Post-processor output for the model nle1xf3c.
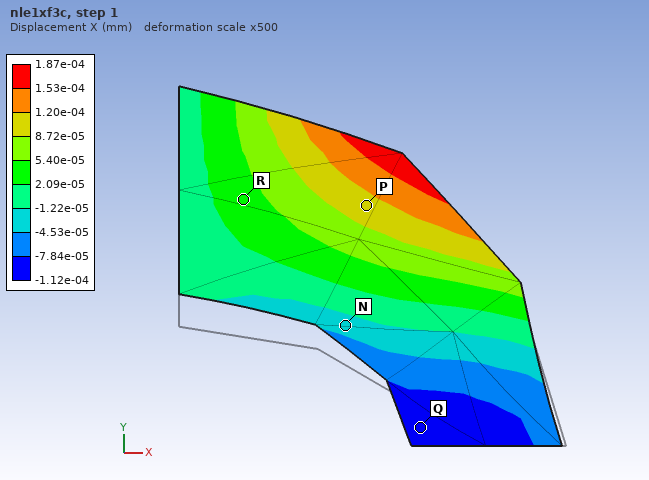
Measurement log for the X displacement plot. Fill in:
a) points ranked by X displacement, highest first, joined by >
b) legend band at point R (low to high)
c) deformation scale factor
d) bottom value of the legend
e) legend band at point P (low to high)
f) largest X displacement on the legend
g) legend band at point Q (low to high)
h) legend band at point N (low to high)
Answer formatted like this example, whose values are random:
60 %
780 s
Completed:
P > R > N > Q
2.09e-05 to 5.40e-05 mm
500
-1.12e-04 mm
8.72e-05 to 1.20e-04 mm
1.87e-04 mm
-1.12e-04 to -7.84e-05 mm
-4.53e-05 to -1.22e-05 mm
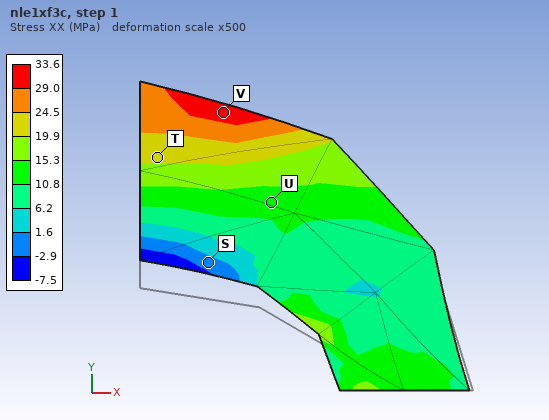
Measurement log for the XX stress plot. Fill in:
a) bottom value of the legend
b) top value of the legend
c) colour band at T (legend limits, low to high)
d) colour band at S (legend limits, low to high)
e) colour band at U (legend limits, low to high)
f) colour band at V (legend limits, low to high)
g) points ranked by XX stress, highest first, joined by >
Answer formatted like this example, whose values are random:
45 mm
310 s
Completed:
-7.5 MPa
33.6 MPa
19.9 to 24.5 MPa
-2.9 to 1.6 MPa
10.8 to 15.3 MPa
29.0 to 33.6 MPa
V > T > U > S
